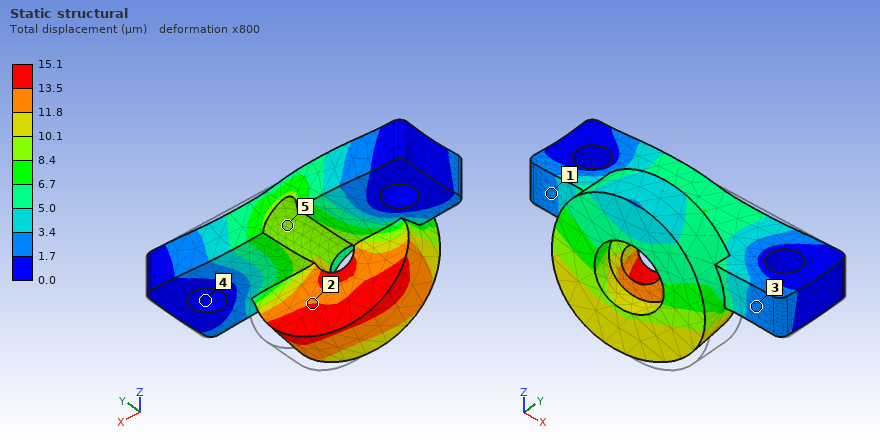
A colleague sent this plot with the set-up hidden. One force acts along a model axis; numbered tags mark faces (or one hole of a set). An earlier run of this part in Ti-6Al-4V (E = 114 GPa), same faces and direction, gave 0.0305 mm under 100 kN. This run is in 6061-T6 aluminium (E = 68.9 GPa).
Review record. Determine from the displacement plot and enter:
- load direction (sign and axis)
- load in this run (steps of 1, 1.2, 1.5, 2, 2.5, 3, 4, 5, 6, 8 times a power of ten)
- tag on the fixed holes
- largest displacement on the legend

-X
30 kN
4
15.1 µm
